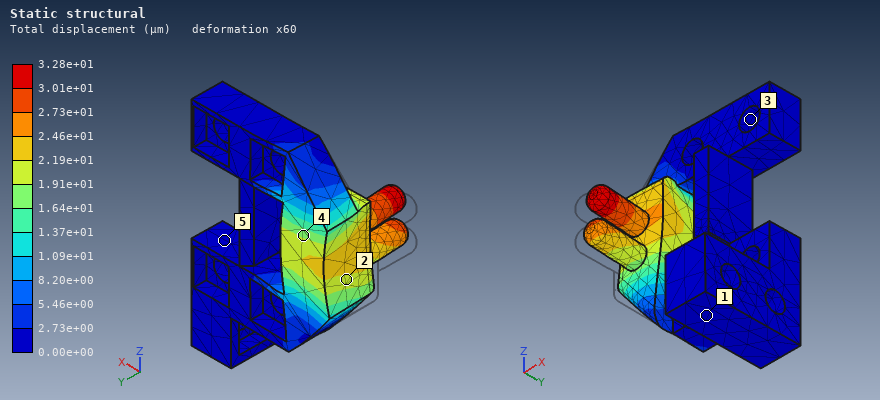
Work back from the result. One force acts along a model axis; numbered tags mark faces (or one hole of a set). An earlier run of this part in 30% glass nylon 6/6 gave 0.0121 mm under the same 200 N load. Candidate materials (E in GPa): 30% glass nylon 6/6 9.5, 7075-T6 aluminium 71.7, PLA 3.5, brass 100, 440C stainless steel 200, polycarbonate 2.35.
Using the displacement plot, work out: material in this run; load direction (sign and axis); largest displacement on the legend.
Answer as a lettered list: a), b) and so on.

a) PLA
b) +X
c) 3.28e+01 µm
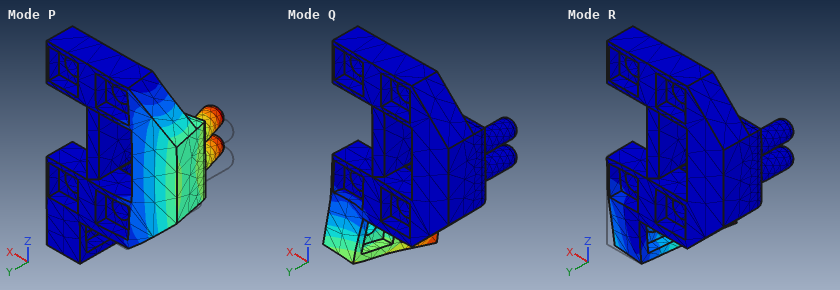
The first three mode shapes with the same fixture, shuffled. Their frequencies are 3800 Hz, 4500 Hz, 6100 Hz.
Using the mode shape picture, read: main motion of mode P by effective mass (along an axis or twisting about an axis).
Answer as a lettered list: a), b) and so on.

a) along Y
